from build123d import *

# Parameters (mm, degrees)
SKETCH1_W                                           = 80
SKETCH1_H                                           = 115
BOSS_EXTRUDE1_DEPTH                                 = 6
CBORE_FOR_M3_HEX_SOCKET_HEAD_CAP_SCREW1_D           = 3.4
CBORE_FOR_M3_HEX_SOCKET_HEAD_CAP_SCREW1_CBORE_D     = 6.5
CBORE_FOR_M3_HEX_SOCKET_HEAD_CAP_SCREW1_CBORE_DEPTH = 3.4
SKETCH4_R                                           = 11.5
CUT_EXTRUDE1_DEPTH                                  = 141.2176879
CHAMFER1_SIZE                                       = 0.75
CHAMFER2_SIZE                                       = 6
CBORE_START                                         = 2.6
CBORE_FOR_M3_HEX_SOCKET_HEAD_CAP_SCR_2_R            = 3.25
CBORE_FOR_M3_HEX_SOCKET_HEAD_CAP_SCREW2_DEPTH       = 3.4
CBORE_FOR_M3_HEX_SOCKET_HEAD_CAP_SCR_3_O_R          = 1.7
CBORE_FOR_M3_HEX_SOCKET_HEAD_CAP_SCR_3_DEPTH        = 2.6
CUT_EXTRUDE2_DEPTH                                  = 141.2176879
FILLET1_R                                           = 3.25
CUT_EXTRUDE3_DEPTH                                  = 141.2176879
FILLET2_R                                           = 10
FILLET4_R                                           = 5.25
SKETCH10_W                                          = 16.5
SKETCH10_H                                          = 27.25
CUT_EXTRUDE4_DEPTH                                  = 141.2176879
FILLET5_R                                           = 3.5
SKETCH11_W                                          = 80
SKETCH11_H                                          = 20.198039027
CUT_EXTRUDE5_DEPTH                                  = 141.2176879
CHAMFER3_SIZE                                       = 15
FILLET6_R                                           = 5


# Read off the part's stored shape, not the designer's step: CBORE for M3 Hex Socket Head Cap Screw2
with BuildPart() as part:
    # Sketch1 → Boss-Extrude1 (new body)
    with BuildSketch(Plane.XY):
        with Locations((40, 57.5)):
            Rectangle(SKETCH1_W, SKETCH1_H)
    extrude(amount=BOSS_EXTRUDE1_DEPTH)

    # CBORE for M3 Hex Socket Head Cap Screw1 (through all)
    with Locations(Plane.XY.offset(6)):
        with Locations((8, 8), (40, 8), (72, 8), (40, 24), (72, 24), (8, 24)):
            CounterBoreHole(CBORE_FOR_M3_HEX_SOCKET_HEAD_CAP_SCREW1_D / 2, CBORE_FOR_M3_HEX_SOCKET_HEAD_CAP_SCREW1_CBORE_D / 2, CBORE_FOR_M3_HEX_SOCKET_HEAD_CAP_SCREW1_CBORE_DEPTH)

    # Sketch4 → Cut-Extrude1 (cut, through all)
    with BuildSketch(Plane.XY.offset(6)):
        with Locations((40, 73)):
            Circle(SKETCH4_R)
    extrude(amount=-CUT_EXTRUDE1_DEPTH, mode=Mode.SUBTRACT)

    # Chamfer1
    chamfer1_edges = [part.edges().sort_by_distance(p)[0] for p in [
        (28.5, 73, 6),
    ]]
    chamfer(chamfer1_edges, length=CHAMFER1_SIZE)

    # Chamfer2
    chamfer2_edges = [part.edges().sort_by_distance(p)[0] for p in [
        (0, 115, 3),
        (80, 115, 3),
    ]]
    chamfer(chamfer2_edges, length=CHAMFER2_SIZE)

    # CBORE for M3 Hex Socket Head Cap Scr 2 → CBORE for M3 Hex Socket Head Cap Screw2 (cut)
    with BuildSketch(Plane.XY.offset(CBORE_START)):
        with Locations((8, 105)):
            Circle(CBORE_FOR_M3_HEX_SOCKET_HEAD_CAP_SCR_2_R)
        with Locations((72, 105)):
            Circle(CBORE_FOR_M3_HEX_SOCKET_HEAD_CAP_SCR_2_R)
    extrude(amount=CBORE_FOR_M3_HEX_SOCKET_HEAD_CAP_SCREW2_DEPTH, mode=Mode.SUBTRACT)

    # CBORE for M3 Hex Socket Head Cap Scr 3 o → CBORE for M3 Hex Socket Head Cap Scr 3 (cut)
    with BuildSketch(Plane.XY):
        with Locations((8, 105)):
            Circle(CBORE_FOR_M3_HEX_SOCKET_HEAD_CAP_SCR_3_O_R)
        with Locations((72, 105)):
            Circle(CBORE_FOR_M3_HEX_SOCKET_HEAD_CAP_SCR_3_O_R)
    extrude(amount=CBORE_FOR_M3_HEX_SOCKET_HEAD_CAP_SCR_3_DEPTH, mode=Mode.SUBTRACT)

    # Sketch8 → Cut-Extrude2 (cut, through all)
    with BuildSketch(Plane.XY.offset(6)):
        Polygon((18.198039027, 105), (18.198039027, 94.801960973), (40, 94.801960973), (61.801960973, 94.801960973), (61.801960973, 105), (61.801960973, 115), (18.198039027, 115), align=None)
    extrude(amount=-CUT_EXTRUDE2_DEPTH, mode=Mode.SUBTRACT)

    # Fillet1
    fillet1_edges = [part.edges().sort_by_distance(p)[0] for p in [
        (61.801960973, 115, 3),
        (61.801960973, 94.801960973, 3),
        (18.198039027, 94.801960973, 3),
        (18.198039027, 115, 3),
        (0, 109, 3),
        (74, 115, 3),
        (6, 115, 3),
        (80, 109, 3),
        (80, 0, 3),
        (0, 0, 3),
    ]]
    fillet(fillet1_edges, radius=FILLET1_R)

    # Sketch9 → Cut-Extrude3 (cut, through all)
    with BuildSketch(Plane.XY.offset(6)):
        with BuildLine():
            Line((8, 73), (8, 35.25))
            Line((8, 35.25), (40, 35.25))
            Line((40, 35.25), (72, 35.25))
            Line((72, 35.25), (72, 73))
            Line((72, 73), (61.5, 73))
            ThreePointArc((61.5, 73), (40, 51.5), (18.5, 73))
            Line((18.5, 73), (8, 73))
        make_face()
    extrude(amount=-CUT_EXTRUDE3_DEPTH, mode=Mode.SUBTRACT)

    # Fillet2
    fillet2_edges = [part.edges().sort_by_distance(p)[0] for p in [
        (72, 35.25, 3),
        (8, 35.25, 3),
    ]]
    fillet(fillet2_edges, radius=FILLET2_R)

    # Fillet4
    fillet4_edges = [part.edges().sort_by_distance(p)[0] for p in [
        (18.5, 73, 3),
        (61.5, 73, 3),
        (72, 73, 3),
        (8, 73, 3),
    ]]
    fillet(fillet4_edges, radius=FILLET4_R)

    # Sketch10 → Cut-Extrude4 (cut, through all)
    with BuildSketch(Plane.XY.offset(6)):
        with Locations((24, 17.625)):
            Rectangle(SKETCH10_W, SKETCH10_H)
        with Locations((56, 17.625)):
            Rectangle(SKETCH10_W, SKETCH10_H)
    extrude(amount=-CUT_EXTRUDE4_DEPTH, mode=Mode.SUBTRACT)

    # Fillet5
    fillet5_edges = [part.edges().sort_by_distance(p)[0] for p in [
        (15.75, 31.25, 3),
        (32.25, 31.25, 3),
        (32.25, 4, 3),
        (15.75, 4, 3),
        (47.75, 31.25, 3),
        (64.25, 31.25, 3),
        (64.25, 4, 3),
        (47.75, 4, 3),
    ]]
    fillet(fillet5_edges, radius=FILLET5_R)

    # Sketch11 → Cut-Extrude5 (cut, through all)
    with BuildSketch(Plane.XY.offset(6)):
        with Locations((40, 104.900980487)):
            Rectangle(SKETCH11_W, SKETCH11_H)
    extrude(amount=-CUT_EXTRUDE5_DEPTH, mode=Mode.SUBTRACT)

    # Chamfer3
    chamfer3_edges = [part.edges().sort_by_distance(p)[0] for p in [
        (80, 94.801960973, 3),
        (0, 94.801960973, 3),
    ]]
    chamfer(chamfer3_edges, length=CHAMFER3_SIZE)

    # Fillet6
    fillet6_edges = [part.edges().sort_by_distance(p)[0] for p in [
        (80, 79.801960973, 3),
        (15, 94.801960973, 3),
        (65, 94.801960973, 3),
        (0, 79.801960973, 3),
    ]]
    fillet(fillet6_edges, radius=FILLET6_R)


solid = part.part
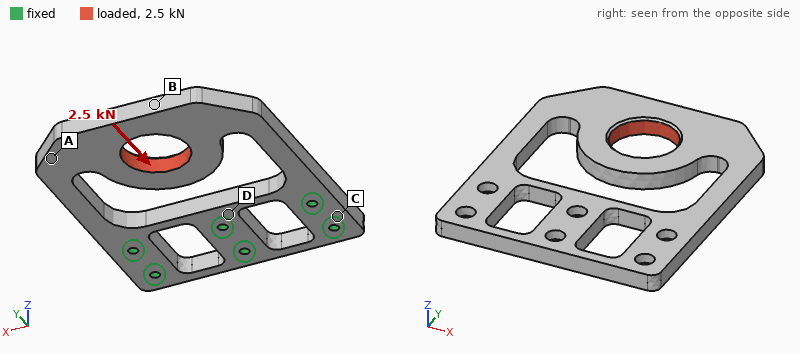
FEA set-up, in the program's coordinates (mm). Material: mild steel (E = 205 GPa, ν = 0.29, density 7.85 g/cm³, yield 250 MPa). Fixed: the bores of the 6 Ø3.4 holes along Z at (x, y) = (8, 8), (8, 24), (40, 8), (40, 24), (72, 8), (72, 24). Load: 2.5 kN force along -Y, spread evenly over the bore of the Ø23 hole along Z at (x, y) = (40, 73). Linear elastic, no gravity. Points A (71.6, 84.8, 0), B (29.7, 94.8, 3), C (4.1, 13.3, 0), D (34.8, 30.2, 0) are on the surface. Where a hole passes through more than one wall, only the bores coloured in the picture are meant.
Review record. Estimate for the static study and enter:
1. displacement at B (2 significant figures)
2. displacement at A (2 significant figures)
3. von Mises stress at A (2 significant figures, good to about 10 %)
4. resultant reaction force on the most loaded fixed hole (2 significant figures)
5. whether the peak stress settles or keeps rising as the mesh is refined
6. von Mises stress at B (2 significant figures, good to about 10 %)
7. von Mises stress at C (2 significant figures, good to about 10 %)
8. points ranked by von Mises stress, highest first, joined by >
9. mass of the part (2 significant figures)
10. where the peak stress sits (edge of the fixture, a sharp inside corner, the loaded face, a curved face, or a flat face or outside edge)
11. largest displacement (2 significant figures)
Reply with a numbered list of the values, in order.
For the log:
1. 29 µm
2. 19 µm
3. 23 MPa
4. 940 N
5. keeps rising
6. 35 MPa
7. 13 MPa
8. B > A > C > D
9. 200 g
10. edge of the fixture
11. 32 µm
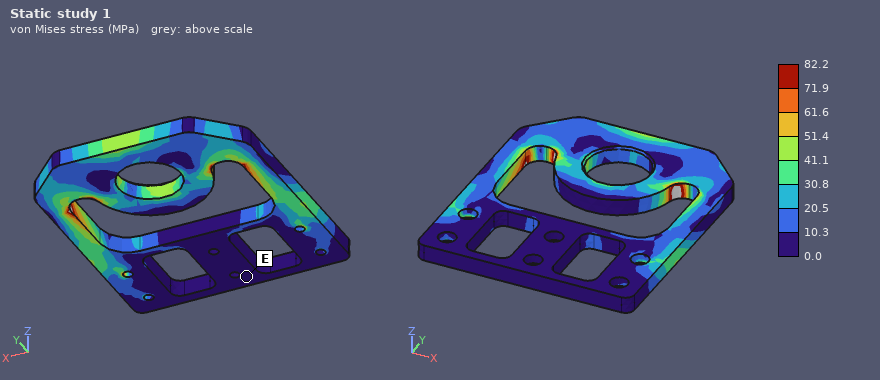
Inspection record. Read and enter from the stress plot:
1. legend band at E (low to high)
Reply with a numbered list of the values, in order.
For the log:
1. 0.0 to 10.3 MPa
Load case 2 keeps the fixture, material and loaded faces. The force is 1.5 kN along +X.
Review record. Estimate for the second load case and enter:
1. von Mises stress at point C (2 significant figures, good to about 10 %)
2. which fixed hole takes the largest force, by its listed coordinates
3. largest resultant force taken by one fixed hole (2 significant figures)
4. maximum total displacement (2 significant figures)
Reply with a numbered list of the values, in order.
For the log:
1. 33 MPa
2. (40, 24)
3. 1.4 kN
4. 0.11 mm
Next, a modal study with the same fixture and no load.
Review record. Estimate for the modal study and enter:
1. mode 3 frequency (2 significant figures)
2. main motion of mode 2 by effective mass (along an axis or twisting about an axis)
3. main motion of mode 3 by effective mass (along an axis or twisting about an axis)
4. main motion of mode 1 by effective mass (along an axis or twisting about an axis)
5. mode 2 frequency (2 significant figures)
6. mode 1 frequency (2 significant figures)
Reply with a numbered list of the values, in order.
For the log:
1. 1900 Hz
2. twisting about Y
3. along X
4. along Z
5. 1600 Hz
6. 570 Hz
